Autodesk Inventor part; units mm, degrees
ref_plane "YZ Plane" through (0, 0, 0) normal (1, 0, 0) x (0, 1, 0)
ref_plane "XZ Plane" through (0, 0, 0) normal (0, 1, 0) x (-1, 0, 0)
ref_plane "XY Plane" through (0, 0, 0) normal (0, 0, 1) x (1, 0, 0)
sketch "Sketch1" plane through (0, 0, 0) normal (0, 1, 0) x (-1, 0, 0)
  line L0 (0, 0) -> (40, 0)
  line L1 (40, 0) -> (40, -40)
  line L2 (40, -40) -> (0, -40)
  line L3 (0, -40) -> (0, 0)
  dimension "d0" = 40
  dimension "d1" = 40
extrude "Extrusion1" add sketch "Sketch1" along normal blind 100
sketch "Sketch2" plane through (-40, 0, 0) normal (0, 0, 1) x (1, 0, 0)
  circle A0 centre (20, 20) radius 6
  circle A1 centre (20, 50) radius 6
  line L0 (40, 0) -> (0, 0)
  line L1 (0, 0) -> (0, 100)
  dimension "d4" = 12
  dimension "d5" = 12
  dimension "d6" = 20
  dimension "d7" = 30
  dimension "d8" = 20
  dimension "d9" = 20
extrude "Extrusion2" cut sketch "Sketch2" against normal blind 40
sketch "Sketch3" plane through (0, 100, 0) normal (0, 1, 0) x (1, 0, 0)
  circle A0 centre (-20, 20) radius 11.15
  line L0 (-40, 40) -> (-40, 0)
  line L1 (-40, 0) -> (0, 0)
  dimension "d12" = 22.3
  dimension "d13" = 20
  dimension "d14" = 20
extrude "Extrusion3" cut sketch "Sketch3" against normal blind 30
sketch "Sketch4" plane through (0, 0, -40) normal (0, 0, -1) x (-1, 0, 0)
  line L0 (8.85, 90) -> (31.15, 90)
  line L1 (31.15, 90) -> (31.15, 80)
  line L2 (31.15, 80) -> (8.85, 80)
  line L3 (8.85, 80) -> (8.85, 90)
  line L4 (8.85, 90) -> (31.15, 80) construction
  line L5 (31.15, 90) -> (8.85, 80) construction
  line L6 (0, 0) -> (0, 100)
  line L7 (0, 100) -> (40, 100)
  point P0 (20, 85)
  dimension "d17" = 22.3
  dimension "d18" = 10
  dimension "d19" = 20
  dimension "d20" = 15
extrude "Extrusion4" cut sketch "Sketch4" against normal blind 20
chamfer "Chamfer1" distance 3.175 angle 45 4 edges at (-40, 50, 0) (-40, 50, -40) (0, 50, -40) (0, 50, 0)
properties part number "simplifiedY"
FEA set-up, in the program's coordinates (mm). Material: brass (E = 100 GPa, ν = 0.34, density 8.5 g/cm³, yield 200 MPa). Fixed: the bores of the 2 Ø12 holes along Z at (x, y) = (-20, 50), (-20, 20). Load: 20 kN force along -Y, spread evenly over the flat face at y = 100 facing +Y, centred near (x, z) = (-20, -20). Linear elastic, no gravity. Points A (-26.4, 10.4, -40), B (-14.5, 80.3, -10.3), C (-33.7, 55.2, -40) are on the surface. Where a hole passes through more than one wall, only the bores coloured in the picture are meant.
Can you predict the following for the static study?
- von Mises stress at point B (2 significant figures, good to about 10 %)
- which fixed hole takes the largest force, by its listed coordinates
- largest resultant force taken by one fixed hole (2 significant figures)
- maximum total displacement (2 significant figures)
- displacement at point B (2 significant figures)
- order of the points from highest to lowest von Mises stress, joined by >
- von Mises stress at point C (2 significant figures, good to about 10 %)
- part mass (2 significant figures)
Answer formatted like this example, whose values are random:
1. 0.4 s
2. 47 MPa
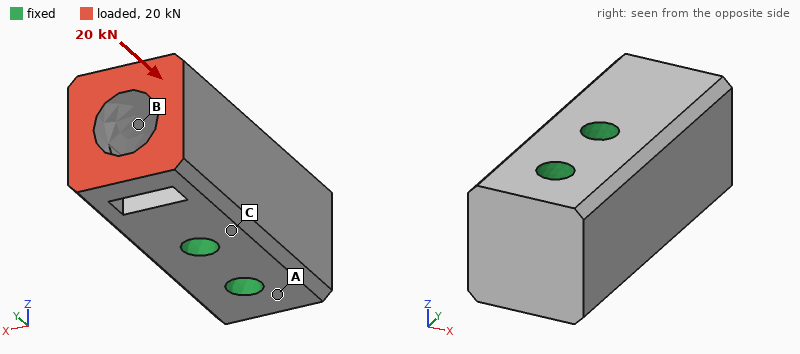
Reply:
1. 23 MPa
2. (-20, 50)
3. 17 kN
4. 25 µm
5. 5.2 µm
6. B > C > A
7. 12 MPa
8. 1.1 kg
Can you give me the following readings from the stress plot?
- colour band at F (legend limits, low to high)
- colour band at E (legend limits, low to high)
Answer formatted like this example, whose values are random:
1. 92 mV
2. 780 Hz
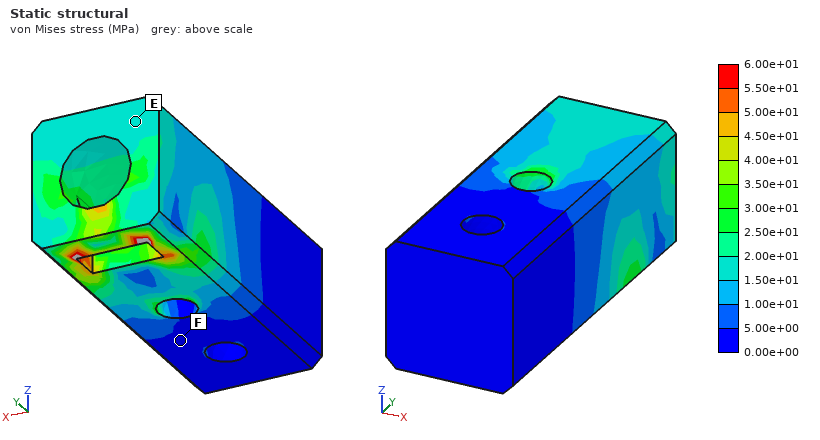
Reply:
1. 0.00e+00 to 5.00e+00 MPa
2. 1.50e+01 to 2.00e+01 MPa
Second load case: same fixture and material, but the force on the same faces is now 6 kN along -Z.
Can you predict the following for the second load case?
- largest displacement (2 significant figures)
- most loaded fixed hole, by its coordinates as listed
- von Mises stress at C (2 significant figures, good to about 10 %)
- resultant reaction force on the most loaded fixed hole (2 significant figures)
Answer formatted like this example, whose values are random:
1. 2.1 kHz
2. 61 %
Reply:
1. 31 µm
2. (-20, 50)
3. 18 MPa
4. 6.9 kN
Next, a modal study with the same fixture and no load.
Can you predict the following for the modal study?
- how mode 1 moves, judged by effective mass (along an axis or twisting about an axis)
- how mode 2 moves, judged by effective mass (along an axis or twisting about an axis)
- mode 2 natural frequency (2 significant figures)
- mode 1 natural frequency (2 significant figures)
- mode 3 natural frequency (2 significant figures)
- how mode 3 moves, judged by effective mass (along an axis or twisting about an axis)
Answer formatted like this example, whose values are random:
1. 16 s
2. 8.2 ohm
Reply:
1. along X
2. along Z
3. 6700 Hz
4. 5500 Hz
5. 9700 Hz
6. twisting about Y
